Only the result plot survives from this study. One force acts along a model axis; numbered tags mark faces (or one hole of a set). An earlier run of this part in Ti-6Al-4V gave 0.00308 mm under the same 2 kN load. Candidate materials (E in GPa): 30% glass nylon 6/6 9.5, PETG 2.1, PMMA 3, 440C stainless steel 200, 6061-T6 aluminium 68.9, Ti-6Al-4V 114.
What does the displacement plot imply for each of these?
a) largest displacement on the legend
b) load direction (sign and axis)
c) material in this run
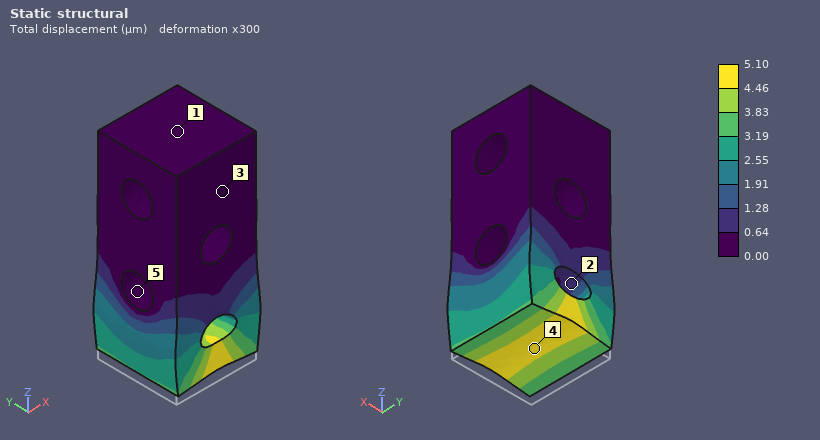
5.10 µm
+Z
6061-T6 aluminium
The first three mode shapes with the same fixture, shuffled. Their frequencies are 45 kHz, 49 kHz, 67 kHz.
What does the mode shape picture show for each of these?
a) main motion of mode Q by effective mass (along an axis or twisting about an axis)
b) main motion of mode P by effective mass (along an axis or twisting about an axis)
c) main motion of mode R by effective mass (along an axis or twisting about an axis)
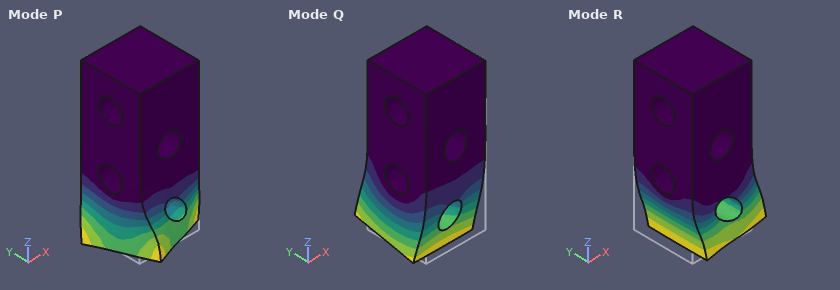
along Y
twisting about Z
along X
